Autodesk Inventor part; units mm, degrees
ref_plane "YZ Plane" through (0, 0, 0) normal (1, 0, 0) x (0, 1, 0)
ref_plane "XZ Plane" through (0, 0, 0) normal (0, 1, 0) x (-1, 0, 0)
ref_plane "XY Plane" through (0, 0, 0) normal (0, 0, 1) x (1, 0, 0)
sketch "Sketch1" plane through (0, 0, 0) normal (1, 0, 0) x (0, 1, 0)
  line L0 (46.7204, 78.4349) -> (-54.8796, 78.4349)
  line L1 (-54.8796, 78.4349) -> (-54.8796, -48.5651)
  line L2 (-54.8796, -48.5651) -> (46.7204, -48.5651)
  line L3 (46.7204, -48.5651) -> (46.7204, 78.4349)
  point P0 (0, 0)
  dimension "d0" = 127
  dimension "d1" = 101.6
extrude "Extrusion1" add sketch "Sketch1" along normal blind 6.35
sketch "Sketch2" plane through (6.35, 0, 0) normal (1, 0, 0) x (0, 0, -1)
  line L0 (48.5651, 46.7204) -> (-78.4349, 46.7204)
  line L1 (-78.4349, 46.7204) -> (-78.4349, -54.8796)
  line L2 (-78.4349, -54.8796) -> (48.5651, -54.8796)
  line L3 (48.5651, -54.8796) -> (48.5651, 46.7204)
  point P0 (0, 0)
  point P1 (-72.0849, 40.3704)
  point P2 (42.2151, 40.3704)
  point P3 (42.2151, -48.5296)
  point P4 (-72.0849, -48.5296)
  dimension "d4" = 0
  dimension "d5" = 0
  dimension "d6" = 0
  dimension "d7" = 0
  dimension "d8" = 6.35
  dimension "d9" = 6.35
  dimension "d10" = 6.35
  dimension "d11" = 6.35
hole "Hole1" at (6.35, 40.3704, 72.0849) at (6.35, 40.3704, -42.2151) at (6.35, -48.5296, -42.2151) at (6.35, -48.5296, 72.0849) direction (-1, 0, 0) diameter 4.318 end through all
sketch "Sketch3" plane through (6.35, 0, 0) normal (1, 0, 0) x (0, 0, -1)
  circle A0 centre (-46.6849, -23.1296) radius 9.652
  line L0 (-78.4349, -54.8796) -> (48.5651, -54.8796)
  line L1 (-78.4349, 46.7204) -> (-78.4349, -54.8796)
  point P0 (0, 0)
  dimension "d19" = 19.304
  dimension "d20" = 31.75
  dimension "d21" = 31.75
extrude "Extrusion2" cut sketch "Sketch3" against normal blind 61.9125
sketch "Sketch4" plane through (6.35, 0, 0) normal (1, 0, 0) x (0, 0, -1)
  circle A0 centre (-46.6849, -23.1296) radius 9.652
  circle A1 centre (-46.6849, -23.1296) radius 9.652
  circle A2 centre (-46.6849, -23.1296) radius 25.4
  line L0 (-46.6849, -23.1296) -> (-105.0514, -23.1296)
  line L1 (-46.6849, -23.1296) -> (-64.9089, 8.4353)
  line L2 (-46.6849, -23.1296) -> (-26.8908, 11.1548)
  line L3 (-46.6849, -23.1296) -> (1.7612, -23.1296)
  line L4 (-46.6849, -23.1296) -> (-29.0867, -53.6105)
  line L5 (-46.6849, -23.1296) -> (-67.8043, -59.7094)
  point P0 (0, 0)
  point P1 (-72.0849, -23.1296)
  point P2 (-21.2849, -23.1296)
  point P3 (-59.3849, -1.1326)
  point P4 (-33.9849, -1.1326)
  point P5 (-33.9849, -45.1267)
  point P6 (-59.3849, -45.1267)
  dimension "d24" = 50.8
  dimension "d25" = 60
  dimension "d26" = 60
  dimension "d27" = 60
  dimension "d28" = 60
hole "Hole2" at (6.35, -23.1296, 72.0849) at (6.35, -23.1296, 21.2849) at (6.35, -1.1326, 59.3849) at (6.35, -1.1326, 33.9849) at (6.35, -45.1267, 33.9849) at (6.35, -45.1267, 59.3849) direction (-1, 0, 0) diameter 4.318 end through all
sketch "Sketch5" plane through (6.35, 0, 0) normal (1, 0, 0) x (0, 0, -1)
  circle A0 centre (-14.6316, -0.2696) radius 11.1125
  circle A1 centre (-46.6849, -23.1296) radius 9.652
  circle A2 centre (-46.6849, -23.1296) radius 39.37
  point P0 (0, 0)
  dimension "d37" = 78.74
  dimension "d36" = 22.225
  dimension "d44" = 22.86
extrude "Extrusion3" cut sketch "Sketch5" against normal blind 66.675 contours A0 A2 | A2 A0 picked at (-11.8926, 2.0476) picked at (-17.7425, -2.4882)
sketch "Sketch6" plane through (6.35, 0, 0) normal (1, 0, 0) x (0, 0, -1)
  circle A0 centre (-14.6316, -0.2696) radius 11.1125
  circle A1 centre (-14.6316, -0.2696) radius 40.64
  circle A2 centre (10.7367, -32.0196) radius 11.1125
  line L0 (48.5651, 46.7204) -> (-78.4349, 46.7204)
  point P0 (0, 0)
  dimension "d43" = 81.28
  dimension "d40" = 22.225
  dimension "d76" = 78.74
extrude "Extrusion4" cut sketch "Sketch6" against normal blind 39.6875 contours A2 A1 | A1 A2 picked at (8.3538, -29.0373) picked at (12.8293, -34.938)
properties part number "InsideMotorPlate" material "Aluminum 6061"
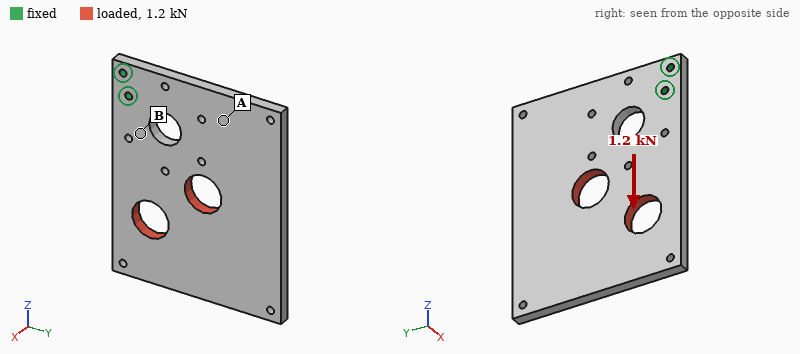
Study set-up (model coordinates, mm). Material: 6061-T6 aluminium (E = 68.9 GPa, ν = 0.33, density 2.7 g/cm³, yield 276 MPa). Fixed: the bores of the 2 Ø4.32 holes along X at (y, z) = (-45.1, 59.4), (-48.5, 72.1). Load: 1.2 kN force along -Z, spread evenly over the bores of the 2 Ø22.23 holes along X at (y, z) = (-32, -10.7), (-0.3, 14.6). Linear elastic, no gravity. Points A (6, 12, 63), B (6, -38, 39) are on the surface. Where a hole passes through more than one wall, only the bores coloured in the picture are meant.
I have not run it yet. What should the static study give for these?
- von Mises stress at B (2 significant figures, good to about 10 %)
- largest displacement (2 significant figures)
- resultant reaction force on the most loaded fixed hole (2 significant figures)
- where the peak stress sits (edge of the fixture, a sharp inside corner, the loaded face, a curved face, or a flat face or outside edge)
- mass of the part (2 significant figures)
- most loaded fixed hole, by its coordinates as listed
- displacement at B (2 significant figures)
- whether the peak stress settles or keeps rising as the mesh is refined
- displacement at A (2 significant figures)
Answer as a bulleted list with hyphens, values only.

- 9.9 MPa
- 0.13 mm
- 2.4 kN
- edge of the fixture
- 200 g
- (-45.1, 59.4)
- 0.021 mm
- keeps rising
- 0.055 mm
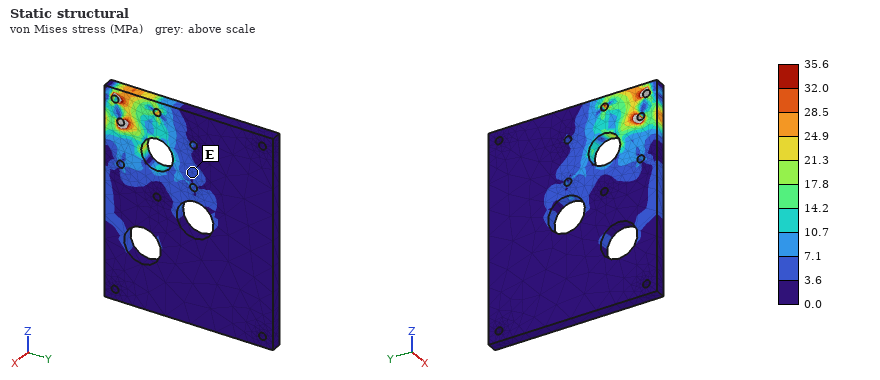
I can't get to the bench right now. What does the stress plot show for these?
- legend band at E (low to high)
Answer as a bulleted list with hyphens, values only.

- 3.6 to 7.1 MPa
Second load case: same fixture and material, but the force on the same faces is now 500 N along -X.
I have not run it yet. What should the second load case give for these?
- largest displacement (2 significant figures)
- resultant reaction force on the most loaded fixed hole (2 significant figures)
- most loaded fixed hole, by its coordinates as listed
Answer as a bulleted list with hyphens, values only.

- 1.9 mm
- 1.5 kN
- (-45.1, 59.4)
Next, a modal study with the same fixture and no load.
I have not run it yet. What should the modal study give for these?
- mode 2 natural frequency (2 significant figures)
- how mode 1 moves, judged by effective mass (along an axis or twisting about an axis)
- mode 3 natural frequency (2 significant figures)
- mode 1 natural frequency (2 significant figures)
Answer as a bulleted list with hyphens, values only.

- 490 Hz
- along X
- 840 Hz
- 240 Hz
